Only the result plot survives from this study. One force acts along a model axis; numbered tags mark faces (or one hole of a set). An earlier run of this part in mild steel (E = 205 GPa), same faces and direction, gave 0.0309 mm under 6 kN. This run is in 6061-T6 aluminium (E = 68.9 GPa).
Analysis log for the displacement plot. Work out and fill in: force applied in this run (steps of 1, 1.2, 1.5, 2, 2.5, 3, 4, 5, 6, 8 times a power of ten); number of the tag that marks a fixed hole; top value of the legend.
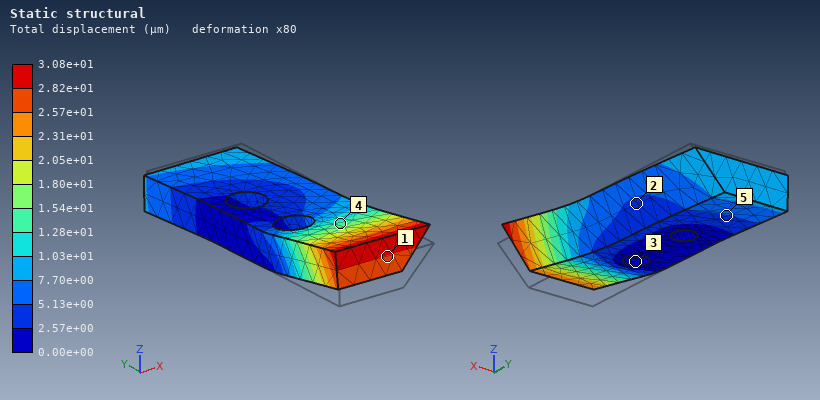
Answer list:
2 kN
3
3.08e+01 µm
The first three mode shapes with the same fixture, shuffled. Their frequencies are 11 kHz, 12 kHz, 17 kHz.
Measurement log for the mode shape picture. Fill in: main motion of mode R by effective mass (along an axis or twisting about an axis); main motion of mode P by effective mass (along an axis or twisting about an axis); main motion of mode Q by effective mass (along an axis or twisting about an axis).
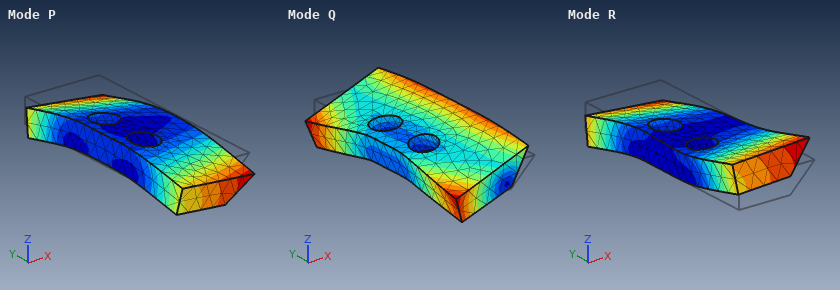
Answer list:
twisting about X
along Z
along X
